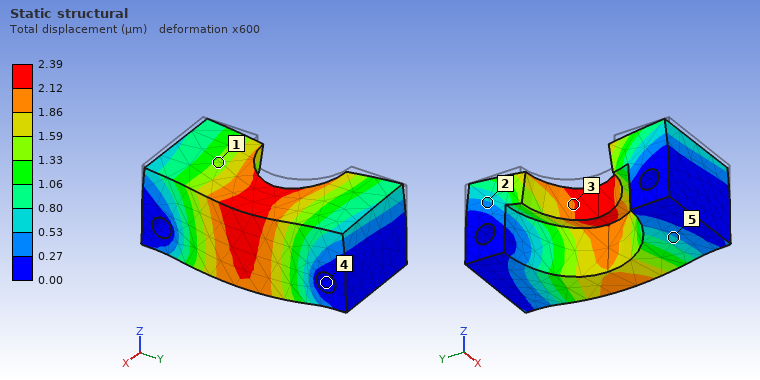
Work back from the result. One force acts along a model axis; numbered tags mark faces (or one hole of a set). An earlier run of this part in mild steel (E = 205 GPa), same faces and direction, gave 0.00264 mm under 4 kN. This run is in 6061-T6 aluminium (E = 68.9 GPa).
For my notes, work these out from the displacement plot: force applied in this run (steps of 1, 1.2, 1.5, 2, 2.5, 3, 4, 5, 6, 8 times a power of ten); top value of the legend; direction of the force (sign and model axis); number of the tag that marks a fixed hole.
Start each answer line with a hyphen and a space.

- 1.2 kN
- 2.39 µm
- -Z
- 4
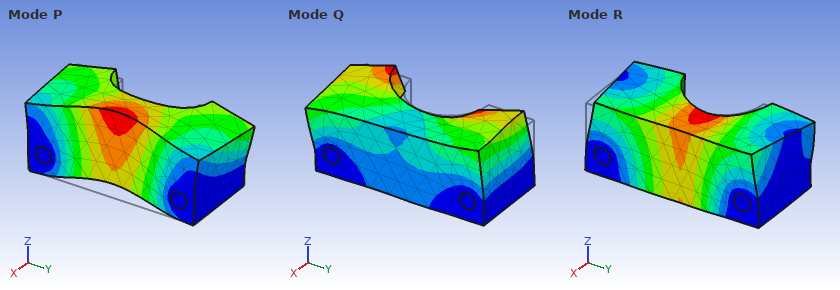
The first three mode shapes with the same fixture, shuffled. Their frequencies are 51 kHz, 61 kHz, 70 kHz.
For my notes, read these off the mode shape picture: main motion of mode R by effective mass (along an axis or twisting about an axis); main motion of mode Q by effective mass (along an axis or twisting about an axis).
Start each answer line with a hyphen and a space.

- along X
- along Y
